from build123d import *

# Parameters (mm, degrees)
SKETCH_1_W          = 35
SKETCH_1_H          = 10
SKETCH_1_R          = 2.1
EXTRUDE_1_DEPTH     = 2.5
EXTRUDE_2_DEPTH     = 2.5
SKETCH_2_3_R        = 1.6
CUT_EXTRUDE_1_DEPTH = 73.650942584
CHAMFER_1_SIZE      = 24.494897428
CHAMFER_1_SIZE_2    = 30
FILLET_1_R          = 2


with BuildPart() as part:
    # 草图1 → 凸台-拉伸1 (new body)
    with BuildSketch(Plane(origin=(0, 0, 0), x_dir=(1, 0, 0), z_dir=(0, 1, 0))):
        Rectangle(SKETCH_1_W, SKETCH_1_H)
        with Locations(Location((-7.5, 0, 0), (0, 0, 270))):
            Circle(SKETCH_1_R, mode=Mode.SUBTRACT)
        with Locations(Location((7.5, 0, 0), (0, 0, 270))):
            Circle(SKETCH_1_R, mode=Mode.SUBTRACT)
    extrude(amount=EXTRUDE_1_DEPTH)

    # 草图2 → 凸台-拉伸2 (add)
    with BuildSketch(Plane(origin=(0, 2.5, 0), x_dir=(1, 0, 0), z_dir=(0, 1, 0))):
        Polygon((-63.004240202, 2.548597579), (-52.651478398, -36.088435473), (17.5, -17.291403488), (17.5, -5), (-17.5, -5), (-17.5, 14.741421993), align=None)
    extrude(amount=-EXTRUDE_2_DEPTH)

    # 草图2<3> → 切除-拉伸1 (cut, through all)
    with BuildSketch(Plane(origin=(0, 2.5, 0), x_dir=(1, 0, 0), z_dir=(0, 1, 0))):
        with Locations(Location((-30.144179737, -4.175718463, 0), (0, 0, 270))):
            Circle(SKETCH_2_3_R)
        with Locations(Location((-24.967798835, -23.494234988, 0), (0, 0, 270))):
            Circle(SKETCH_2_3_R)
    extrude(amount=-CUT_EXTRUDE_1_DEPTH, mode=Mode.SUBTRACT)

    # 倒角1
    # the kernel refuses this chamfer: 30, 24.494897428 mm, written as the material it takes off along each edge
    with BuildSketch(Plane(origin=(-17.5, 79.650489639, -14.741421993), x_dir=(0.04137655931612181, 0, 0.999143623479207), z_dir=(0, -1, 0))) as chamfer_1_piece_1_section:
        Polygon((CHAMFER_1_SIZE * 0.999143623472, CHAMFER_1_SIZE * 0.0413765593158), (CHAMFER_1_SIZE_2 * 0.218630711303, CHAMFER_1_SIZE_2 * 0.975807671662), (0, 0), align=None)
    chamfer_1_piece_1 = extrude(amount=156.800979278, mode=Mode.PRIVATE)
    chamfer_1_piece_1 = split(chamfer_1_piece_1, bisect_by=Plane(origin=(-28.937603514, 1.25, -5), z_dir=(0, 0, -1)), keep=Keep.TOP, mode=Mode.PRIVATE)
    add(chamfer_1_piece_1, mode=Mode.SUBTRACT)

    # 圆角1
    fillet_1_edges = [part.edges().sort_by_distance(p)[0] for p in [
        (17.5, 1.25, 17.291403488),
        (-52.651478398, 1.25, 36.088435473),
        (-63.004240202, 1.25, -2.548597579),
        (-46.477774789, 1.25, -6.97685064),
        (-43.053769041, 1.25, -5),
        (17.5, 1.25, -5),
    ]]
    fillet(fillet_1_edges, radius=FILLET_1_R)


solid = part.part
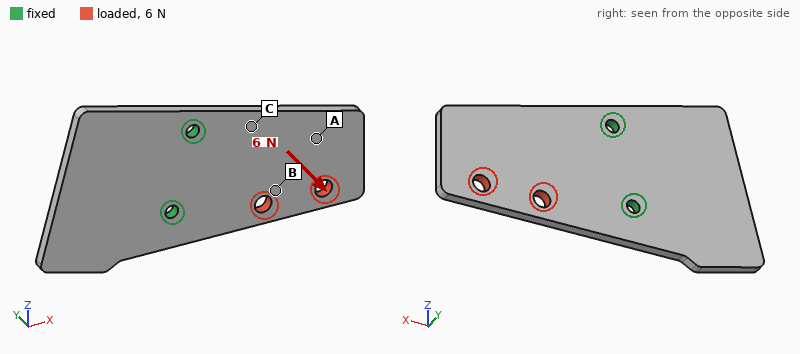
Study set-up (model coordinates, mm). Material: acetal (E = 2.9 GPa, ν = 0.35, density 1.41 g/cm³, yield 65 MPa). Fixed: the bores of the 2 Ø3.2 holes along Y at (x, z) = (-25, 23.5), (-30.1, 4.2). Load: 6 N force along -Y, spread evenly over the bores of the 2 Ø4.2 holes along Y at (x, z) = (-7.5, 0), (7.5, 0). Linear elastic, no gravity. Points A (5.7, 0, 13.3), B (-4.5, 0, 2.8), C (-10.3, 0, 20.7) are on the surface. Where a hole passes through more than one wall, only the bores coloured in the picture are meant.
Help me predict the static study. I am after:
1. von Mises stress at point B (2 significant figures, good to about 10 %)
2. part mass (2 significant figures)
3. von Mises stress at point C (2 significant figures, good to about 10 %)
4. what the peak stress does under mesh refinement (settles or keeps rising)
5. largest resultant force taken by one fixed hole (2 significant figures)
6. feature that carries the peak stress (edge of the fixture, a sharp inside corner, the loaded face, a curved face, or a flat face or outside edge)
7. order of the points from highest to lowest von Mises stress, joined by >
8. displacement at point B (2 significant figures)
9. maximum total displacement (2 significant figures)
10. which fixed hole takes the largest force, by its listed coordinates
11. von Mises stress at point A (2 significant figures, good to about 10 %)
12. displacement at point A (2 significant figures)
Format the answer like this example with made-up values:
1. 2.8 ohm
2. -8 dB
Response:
1. 1.7 MPa
2. 8.5 g
3. 2.8 MPa
4. keeps rising
5. 4.6 N
6. edge of the fixture
7. C > B > A
8. 0.35 mm
9. 0.91 mm
10. (-30.1, 4.2)
11. 0.82 MPa
12. 0.47 mm
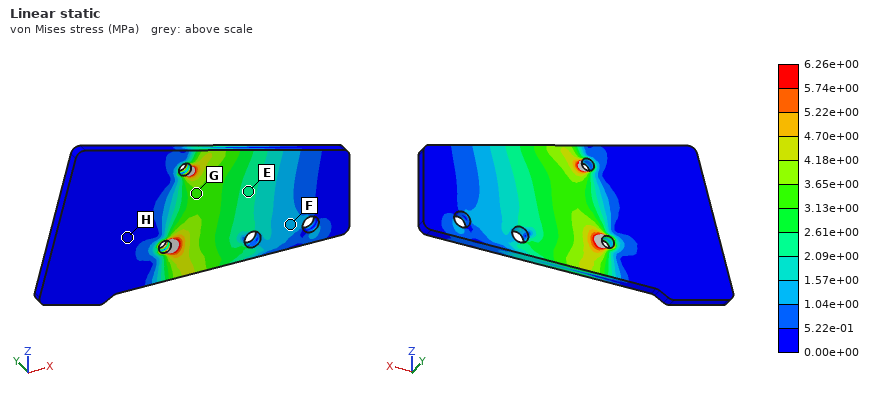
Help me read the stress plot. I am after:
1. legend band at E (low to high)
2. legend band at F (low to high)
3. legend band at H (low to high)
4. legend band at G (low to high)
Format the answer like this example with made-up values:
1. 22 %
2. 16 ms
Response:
1. 2.09e+00 to 2.61e+00 MPa
2. 1.04e+00 to 1.57e+00 MPa
3. 0.00e+00 to 5.22e-01 MPa
4. 3.13e+00 to 3.65e+00 MPa
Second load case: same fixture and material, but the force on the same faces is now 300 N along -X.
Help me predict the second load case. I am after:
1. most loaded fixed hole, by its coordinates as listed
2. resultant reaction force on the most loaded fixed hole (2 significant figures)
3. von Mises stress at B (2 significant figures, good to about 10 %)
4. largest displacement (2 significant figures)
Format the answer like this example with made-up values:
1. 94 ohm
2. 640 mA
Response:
1. (-30.1, 4.2)
2. 350 N
3. 8.1 MPa
4. 0.26 mm
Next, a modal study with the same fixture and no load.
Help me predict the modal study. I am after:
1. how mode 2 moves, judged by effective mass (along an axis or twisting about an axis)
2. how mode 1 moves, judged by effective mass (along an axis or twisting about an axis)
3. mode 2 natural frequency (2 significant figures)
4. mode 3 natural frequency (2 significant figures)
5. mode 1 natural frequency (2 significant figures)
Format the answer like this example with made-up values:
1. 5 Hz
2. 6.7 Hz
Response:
1. along Y
2. along Y
3. 610 Hz
4. 1100 Hz
5. 320 Hz
